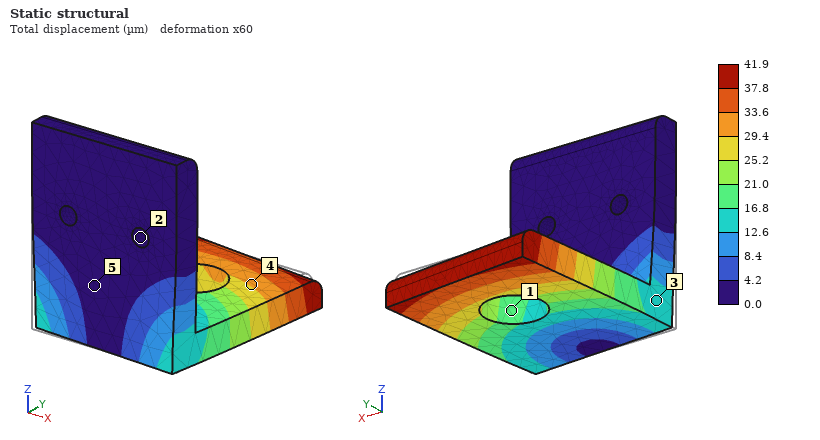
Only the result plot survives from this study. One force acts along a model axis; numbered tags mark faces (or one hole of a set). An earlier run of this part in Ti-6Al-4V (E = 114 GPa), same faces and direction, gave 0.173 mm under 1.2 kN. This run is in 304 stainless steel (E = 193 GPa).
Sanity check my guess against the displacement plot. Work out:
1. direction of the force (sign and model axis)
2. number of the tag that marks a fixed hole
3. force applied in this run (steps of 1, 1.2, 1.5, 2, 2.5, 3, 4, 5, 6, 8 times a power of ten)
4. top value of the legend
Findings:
+X
2
500 N
41.9 µm
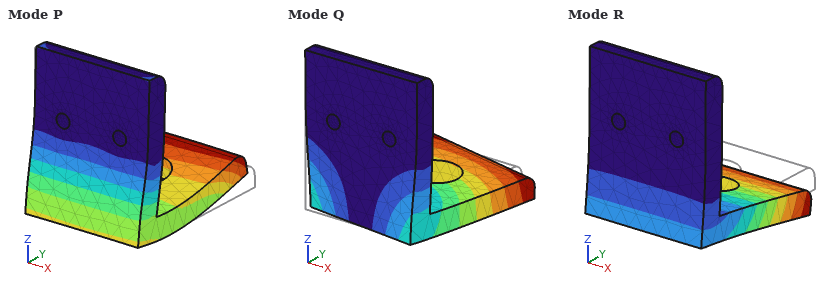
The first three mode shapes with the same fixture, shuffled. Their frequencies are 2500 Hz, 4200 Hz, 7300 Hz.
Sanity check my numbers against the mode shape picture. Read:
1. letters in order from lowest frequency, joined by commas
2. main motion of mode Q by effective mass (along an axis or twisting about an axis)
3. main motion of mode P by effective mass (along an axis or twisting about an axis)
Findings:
R, Q, P
along X
along Y
